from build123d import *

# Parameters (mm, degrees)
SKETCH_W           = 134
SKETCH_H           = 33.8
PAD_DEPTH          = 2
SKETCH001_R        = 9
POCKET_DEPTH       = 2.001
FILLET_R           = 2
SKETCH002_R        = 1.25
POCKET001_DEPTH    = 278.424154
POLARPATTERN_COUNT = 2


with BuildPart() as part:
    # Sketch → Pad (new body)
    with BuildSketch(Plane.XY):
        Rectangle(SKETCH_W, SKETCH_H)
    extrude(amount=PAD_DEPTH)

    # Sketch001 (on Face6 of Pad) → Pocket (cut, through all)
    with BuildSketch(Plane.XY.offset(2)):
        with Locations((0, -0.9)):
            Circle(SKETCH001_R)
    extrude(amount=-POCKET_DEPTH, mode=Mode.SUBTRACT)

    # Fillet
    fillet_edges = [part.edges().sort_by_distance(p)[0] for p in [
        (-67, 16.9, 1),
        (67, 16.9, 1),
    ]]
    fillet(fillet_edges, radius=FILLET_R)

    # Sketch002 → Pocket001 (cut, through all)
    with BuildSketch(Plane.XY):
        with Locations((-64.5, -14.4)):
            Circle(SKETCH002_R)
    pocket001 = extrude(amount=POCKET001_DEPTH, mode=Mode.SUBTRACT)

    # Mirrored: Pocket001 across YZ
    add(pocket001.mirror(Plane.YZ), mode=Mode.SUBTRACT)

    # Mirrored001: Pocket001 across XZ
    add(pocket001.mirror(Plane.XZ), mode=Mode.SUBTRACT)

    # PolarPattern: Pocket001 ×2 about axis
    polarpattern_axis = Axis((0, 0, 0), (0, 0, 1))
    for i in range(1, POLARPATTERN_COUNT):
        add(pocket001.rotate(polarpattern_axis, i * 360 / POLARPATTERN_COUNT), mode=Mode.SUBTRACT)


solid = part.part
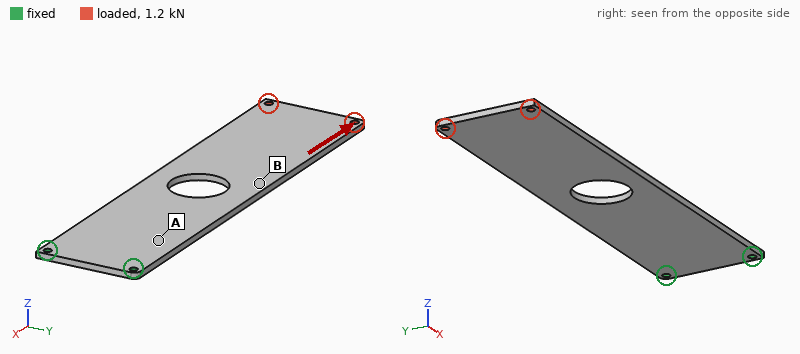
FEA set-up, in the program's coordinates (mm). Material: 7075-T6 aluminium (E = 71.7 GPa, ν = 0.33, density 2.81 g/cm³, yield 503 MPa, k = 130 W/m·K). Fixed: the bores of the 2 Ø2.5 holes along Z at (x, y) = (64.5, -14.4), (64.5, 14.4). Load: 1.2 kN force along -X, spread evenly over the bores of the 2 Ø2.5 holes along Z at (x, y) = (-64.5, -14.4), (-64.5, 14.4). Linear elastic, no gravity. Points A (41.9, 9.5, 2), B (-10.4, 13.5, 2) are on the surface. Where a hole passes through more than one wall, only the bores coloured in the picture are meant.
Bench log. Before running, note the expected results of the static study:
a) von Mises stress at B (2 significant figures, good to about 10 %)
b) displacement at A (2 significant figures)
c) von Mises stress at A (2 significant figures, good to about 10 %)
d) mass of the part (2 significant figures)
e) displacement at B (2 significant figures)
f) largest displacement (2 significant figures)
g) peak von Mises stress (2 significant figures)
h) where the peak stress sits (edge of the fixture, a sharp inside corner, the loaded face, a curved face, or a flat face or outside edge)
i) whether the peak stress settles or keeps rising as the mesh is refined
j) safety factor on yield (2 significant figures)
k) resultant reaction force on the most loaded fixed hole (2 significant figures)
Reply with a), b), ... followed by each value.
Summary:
a) 30 MPa
b) 8.9 µm
c) 18 MPa
d) 24 g
e) 27 µm
f) 54 µm
g) 150 MPa
h) the loaded face
i) settles
j) 3.3
k) 630 N
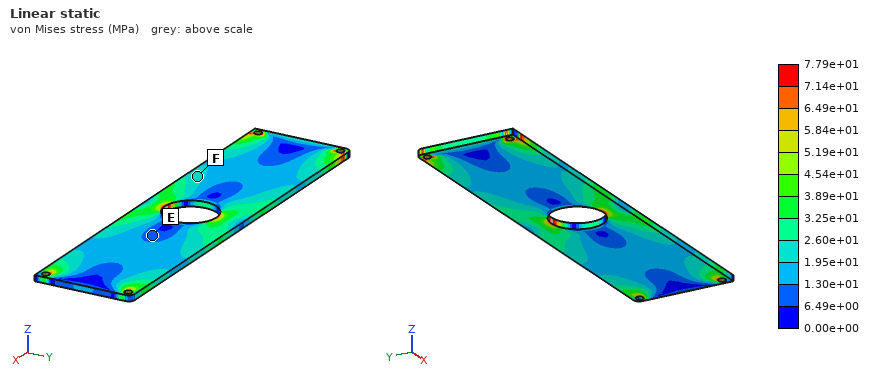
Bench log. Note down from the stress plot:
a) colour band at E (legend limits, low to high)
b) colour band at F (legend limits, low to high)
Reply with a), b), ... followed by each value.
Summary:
a) 6.49e+00 to 1.30e+01 MPa
b) 1.95e+01 to 2.60e+01 MPa
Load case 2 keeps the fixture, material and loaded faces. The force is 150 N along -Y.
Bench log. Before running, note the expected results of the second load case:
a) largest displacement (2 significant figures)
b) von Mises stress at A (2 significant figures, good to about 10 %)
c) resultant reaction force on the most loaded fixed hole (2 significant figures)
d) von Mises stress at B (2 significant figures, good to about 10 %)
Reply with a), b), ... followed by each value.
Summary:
a) 0.28 mm
b) 24 MPa
c) 680 N
d) 15 MPa
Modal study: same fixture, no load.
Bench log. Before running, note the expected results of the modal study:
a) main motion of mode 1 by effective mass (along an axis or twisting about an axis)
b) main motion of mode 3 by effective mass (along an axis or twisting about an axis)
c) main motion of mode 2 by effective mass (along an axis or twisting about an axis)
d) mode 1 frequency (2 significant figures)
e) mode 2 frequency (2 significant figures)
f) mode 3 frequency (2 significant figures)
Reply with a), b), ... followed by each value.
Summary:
a) along Z
b) twisting about X
c) along Z
d) 89 Hz
e) 540 Hz
f) 700 Hz
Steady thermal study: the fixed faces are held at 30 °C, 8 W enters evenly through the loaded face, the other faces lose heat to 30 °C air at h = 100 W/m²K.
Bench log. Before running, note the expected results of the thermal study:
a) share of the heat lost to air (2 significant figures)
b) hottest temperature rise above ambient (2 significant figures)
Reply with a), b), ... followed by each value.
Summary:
a) 97 %
b) 39 K
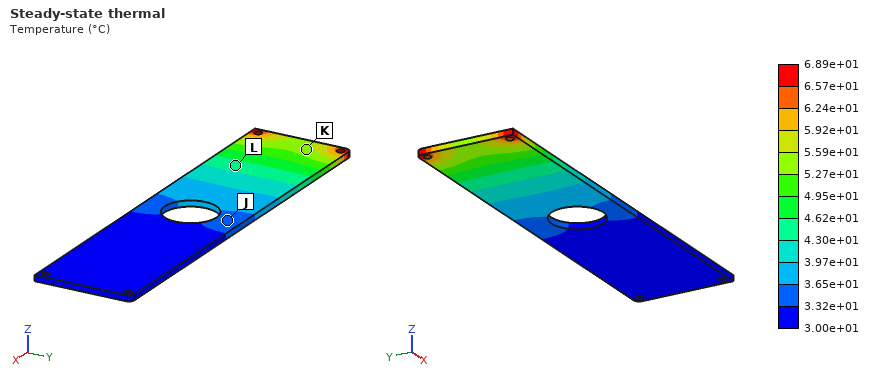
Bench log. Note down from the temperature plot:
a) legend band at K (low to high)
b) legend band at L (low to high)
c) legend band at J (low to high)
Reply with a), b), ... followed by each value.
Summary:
a) 5.27e+01 to 5.59e+01 °C
b) 4.30e+01 to 4.62e+01 °C
c) 3.32e+01 to 3.65e+01 °C
